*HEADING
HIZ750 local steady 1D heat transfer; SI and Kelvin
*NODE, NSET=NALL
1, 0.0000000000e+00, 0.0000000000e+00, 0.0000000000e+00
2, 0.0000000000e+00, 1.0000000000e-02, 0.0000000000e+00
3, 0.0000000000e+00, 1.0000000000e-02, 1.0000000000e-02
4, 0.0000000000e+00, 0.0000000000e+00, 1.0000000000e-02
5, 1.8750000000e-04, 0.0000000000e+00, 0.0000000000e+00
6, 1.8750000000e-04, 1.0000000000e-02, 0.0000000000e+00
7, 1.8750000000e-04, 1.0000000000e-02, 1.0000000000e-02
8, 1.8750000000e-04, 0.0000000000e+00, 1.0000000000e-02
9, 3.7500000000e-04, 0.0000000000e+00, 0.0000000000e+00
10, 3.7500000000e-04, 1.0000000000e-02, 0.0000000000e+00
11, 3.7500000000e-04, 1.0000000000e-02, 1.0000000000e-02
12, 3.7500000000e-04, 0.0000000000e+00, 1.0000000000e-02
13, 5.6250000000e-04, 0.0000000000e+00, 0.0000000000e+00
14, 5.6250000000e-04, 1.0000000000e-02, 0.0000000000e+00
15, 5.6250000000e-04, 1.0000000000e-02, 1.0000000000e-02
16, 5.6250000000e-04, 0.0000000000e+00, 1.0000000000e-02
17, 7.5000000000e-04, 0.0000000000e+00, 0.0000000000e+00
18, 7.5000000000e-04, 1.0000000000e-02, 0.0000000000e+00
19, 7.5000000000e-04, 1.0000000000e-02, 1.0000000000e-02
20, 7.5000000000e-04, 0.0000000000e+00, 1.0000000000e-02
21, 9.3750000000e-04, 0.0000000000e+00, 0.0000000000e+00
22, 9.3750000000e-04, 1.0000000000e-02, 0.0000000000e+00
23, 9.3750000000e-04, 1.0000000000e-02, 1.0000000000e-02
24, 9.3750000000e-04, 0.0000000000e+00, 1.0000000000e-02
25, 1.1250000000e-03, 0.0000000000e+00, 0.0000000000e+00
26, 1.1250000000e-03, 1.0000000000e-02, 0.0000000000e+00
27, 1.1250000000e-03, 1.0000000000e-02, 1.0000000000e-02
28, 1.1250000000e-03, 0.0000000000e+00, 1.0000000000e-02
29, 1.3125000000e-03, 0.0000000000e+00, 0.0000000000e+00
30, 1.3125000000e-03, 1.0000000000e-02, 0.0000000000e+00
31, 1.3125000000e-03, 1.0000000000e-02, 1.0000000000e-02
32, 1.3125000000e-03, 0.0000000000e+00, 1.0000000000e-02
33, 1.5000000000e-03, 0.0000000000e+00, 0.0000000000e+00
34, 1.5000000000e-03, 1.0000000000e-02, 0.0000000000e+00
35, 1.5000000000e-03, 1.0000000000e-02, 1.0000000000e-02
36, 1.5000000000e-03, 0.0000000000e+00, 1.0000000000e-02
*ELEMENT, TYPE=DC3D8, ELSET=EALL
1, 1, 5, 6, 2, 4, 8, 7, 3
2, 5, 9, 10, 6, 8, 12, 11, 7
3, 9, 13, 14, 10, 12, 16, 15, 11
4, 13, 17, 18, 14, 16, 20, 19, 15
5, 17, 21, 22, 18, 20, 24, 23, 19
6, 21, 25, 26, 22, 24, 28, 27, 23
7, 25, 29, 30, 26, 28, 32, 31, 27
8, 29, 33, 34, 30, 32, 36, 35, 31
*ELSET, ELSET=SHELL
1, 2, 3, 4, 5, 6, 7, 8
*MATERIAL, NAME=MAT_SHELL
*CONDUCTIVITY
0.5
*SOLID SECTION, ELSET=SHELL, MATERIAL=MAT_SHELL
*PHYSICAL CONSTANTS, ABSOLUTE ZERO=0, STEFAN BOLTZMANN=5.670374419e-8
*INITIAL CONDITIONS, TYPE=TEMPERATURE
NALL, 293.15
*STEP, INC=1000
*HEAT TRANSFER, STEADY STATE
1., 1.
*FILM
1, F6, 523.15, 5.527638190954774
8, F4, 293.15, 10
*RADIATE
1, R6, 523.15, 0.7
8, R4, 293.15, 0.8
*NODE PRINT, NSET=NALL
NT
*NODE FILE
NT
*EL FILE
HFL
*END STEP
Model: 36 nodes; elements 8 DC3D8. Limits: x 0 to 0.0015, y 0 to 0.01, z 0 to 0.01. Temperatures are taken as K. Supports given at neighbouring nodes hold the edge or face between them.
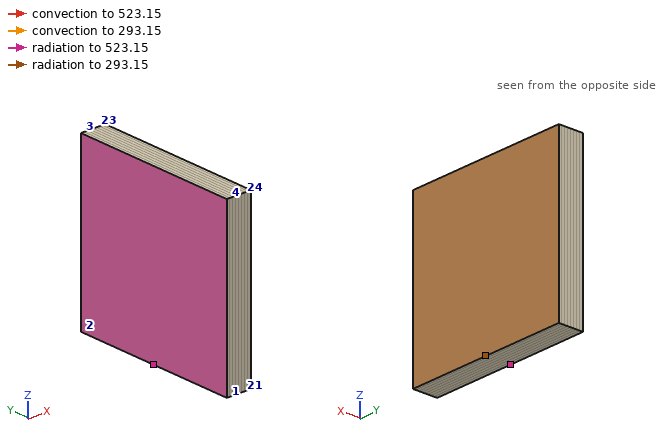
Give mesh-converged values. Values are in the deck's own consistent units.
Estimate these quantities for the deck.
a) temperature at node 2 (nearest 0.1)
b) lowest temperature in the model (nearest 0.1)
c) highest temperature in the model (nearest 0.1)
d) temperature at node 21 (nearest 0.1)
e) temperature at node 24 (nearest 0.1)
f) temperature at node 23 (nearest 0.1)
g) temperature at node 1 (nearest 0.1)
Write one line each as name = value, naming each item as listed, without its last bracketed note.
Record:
temperature at node 2 = 423.0 K
lowest temperature in the model = 416.2 K
highest temperature in the model = 423.0 K
temperature at node 21 = 418.7 K
temperature at node 24 = 418.7 K
temperature at node 23 = 418.7 K
temperature at node 1 = 423.0 K
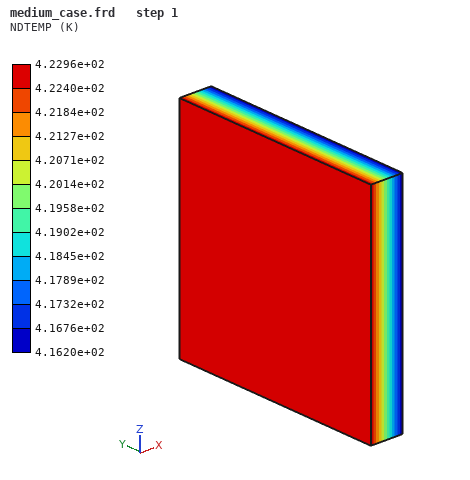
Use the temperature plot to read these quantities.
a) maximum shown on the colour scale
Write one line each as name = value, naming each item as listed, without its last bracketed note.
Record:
maximum shown on the colour scale = 4.2296e+02 K
